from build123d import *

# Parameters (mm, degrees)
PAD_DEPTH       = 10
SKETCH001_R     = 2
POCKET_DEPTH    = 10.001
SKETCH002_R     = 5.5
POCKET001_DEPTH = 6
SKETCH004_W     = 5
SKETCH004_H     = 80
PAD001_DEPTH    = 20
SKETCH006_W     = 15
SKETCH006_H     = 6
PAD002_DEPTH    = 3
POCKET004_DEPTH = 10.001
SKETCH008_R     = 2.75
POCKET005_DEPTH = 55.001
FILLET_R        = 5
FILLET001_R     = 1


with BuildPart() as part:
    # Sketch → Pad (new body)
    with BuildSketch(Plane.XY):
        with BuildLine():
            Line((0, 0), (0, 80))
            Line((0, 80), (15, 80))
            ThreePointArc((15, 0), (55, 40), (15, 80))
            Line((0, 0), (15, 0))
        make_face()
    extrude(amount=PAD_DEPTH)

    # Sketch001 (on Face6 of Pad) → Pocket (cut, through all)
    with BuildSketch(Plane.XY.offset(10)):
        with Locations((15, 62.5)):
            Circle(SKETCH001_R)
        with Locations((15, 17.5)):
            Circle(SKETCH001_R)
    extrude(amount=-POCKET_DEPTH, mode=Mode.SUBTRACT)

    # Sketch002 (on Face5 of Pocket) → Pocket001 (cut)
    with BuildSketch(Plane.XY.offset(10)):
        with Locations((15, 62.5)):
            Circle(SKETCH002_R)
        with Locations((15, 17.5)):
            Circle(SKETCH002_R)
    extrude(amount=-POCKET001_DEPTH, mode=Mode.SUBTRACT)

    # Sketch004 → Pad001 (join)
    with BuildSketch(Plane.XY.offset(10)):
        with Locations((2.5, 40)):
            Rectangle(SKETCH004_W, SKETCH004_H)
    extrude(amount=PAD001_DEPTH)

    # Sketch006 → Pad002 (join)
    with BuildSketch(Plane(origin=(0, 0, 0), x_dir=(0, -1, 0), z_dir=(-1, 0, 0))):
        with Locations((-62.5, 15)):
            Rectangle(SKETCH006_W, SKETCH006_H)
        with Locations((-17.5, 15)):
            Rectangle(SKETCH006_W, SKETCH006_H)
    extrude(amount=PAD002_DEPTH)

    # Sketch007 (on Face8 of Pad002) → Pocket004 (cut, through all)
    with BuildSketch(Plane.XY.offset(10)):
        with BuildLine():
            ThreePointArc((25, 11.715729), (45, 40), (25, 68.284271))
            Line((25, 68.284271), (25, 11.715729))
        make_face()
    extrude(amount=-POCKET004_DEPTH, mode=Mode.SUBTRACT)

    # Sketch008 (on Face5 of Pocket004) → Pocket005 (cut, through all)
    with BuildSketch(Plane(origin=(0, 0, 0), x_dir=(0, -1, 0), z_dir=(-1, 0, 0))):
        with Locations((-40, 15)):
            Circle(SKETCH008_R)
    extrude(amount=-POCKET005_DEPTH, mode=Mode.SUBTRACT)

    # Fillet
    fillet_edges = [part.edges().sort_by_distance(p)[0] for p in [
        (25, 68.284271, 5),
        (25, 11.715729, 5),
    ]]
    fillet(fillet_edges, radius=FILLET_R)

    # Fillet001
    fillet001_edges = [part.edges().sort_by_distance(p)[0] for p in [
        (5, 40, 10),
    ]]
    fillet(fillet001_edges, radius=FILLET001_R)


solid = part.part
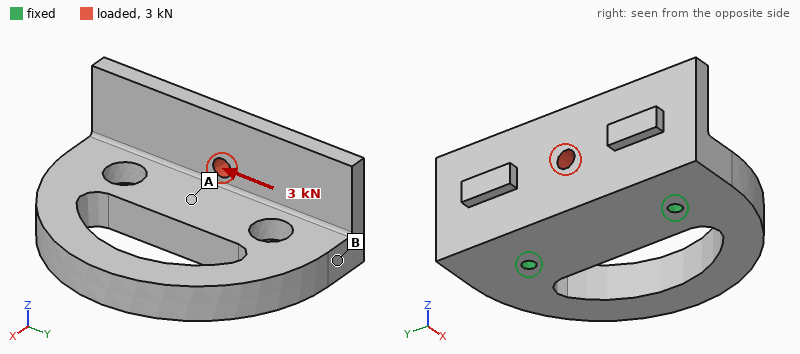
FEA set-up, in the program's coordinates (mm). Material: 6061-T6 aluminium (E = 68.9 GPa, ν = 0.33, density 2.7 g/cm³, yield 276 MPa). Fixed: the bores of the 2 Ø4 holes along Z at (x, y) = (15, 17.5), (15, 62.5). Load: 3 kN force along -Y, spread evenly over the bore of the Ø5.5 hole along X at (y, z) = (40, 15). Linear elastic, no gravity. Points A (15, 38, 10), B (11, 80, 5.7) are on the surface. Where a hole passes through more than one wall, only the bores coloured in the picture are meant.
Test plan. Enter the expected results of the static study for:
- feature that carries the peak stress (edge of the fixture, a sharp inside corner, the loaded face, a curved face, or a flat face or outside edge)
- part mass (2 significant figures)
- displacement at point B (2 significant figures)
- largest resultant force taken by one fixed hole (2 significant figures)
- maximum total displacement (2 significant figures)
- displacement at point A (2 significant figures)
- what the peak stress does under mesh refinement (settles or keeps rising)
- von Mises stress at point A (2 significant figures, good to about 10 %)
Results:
edge of the fixture
98 g
12 µm
1.9 kN
25 µm
3.9 µm
keeps rising
12 MPa
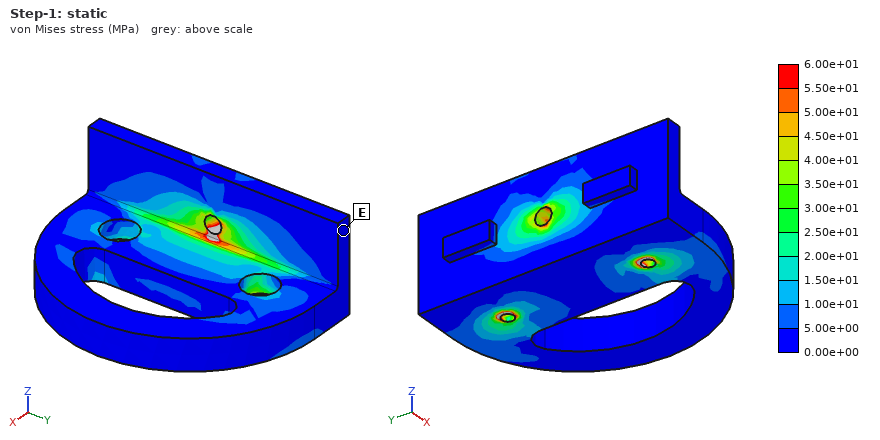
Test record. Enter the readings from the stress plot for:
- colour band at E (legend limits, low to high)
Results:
0.00e+00 to 5.00e+00 MPa
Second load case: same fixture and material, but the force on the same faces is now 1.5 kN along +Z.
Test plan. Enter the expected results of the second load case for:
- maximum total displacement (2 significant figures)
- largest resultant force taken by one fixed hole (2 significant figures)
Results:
93 µm
800 N
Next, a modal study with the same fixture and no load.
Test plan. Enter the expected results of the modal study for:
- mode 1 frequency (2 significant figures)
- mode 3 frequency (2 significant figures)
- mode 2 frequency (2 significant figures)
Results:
2100 Hz
5500 Hz
5000 Hz
